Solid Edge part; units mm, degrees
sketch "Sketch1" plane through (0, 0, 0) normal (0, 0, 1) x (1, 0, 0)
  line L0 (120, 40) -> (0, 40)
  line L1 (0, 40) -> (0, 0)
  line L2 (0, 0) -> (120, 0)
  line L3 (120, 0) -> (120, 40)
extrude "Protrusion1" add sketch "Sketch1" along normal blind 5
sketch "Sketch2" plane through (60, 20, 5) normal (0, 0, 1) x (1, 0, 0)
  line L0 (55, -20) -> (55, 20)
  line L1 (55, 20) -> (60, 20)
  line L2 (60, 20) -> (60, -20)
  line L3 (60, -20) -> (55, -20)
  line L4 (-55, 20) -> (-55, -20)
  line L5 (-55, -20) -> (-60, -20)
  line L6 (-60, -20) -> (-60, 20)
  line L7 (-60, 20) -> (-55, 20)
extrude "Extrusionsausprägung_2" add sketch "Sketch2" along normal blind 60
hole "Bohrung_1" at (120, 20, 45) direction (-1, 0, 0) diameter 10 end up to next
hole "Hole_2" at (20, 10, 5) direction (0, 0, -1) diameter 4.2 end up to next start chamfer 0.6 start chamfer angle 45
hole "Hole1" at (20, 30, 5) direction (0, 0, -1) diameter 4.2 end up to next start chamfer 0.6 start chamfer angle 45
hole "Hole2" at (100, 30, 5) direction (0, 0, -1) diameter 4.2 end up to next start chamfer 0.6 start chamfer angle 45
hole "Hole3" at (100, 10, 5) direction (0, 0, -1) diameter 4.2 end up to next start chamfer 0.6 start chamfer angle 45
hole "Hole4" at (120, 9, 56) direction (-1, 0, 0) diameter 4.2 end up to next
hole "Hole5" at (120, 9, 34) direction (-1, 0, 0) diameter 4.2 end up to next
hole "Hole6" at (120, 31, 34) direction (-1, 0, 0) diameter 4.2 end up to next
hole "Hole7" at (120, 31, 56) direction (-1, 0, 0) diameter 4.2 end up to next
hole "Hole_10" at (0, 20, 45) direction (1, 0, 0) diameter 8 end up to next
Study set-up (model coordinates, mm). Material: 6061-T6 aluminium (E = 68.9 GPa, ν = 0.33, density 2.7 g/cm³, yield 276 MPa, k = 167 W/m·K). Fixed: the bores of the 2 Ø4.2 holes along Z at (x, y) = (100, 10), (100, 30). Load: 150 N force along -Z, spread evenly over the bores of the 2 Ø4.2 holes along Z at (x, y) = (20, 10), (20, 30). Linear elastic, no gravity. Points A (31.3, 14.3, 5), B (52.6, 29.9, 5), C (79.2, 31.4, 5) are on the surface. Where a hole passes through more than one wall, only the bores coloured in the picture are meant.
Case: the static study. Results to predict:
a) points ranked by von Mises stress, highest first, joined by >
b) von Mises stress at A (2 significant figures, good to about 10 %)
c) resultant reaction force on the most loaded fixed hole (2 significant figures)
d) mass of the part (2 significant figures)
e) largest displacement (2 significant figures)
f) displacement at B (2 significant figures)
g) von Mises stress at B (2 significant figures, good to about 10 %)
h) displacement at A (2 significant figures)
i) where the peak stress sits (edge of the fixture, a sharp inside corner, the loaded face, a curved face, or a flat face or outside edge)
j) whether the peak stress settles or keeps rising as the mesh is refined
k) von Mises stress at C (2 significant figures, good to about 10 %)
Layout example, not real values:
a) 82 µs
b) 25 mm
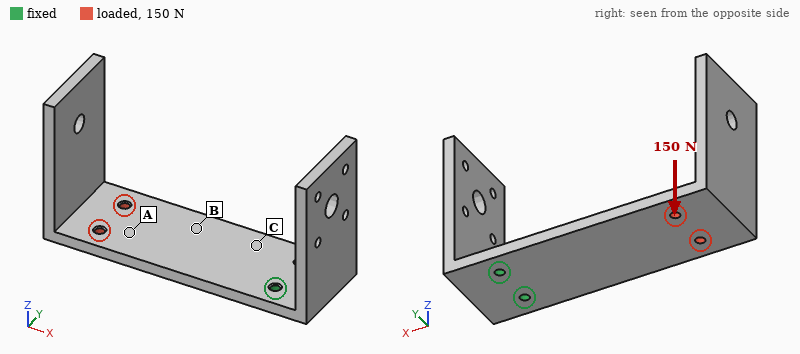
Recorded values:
a) C > B > A
b) 11 MPa
c) 76 N
d) 130 g
e) 1.6 mm
f) 0.38 mm
g) 29 MPa
h) 0.70 mm
i) edge of the fixture
j) keeps rising
k) 51 MPa
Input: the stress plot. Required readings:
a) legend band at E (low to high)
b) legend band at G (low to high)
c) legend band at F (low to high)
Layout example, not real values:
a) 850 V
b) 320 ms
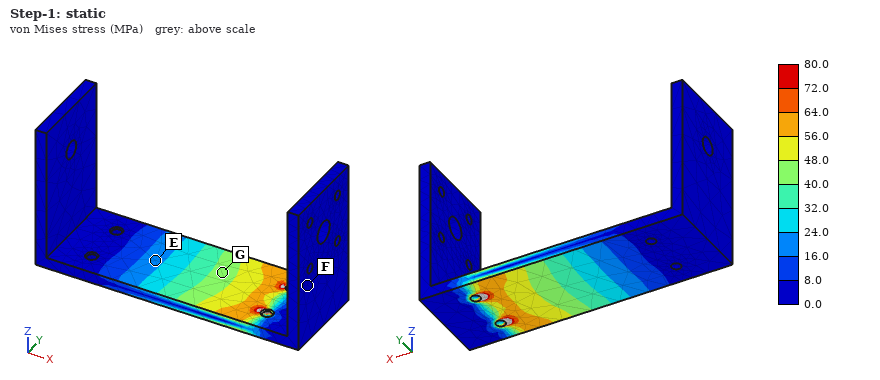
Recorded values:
a) 16.0 to 24.0 MPa
b) 40.0 to 48.0 MPa
c) 0.0 to 8.0 MPa
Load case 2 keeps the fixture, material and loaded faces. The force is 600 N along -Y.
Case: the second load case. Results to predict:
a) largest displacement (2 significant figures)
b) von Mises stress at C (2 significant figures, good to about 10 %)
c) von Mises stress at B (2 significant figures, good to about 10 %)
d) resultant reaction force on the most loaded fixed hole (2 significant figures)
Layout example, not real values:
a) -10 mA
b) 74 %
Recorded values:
a) 0.11 mm
b) 16 MPa
c) 8.8 MPa
d) 2.2 kN
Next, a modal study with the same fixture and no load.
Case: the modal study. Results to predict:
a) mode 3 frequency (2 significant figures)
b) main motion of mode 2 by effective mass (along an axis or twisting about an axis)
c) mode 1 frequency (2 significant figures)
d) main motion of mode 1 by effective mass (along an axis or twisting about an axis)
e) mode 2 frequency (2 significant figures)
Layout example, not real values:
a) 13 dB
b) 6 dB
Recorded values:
a) 700 Hz
b) along Y
c) 210 Hz
d) along Z
e) 480 Hz
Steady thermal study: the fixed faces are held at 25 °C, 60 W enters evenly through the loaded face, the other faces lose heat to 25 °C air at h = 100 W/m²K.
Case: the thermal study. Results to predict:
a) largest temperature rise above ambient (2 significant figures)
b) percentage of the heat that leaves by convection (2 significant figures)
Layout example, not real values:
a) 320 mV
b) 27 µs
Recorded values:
a) 57 K
b) 73 %
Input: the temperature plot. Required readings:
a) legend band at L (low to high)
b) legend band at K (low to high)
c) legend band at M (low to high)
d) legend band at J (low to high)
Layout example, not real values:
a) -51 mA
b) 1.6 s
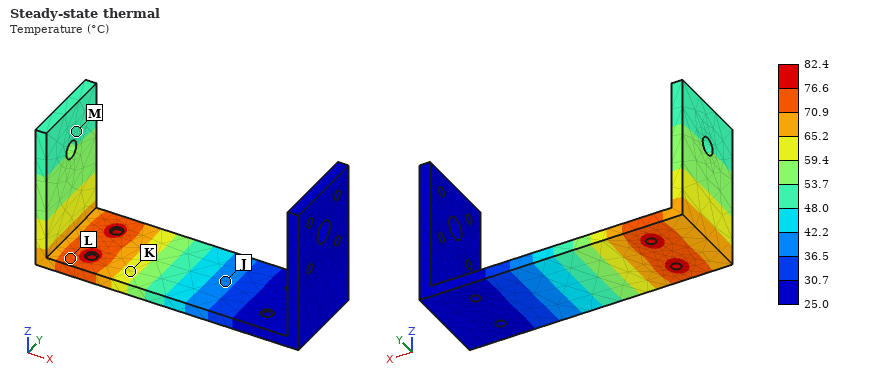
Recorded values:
a) 70.9 to 76.6 °C
b) 59.4 to 65.2 °C
c) 48.0 to 53.7 °C
d) 36.5 to 42.2 °C
